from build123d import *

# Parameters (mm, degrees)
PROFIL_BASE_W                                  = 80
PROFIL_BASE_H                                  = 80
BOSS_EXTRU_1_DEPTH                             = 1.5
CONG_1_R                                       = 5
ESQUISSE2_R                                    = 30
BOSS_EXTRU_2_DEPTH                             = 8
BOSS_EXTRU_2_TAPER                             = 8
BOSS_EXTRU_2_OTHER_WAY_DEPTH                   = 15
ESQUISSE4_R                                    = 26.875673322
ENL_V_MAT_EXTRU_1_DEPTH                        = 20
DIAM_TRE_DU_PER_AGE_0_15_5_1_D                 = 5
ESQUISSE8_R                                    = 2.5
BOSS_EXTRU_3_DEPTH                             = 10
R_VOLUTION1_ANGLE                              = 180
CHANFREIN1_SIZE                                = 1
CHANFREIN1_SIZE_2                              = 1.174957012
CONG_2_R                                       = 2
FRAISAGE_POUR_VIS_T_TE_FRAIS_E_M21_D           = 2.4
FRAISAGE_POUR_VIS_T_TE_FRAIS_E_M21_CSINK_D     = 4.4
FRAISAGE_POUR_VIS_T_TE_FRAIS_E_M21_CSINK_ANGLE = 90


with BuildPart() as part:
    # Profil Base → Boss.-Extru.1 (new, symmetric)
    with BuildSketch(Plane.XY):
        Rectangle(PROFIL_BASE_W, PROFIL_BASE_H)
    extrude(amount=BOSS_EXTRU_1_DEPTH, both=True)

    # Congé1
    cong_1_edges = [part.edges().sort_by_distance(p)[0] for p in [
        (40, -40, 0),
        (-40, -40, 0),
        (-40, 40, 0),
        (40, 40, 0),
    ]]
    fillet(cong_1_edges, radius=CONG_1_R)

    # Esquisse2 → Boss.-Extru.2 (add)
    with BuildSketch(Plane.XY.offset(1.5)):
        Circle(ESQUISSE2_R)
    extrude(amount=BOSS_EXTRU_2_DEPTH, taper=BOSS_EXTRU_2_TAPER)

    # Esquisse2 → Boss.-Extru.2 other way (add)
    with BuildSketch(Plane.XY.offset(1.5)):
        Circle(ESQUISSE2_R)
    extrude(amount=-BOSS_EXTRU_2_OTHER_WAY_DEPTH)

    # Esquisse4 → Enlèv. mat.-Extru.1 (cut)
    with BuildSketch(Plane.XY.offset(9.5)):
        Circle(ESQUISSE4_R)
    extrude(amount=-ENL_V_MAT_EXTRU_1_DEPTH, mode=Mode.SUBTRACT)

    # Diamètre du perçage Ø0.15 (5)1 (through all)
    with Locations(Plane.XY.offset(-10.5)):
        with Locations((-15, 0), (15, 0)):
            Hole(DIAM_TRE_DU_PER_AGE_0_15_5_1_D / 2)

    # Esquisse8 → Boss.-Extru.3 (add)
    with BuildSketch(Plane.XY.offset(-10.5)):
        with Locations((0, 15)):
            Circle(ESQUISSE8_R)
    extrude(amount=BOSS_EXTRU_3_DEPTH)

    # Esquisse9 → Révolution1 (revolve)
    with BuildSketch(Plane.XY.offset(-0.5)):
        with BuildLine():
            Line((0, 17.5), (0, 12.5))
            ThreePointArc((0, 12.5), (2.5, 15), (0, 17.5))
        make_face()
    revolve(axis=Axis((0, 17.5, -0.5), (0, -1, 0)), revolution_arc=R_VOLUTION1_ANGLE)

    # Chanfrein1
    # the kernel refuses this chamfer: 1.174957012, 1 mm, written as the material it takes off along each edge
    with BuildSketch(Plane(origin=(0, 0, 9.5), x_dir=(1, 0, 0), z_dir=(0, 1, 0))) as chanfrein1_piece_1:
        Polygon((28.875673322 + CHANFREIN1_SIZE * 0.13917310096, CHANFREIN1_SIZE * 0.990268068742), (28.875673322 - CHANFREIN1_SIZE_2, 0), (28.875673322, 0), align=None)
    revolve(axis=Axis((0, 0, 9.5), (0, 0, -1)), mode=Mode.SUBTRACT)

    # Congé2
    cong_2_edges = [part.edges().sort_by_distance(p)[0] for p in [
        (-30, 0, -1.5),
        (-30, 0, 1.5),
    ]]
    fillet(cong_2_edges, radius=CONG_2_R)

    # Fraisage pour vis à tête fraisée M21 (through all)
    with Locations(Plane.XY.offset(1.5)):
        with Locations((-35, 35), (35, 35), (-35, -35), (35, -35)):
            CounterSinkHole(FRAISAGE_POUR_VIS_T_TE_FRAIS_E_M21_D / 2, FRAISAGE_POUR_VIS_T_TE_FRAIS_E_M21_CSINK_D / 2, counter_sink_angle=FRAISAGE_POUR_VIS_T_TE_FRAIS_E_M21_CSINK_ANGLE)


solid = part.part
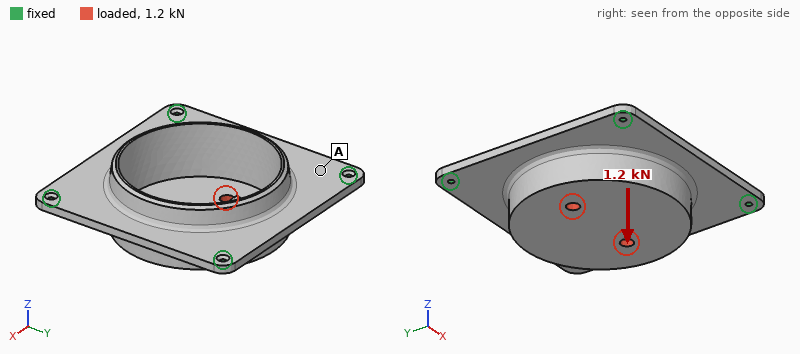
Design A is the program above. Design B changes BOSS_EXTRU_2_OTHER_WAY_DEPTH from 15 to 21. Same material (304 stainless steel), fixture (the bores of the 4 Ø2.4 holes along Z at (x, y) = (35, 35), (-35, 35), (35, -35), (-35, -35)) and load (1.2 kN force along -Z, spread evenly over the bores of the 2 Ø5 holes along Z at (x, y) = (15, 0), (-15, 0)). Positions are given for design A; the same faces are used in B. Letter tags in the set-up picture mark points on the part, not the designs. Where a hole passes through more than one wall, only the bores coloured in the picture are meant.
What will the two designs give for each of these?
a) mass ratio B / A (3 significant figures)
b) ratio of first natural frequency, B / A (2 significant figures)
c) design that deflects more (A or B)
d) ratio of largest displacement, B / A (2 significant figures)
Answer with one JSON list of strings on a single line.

["1.56", "0.78", "A", "0.65"]
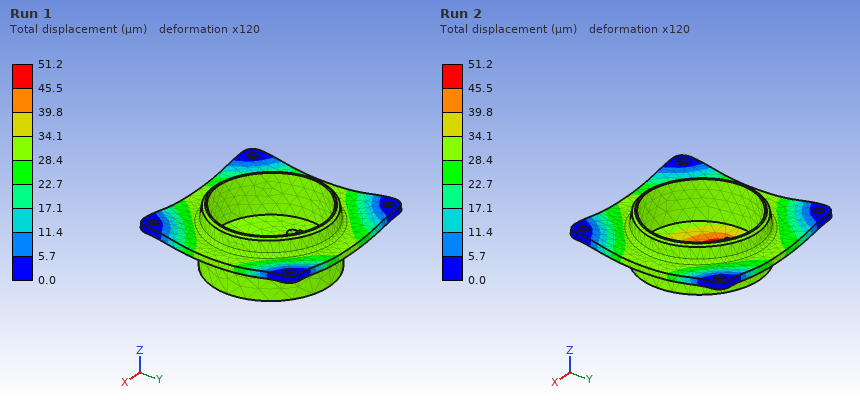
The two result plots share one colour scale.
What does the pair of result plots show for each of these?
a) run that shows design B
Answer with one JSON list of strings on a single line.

["Run 1"]
